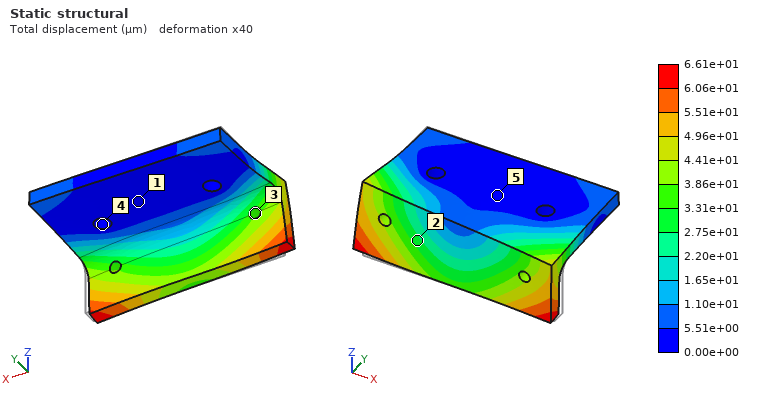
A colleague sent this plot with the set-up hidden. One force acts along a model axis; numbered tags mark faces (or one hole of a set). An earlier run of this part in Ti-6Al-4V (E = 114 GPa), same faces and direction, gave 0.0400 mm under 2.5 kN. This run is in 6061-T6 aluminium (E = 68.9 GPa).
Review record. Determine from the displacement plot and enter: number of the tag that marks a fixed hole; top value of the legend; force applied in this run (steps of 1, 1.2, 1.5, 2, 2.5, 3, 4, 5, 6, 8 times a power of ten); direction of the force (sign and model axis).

4
6.61e+01 µm
2.5 kN
-X
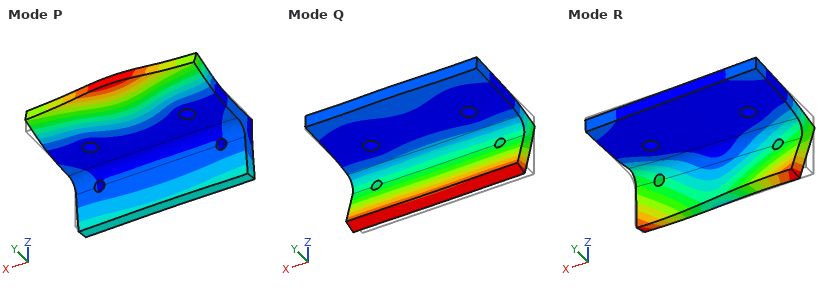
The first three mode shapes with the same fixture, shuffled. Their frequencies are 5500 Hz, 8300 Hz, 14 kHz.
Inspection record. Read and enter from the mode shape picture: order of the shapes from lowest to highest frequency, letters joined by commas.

Q, R, P
